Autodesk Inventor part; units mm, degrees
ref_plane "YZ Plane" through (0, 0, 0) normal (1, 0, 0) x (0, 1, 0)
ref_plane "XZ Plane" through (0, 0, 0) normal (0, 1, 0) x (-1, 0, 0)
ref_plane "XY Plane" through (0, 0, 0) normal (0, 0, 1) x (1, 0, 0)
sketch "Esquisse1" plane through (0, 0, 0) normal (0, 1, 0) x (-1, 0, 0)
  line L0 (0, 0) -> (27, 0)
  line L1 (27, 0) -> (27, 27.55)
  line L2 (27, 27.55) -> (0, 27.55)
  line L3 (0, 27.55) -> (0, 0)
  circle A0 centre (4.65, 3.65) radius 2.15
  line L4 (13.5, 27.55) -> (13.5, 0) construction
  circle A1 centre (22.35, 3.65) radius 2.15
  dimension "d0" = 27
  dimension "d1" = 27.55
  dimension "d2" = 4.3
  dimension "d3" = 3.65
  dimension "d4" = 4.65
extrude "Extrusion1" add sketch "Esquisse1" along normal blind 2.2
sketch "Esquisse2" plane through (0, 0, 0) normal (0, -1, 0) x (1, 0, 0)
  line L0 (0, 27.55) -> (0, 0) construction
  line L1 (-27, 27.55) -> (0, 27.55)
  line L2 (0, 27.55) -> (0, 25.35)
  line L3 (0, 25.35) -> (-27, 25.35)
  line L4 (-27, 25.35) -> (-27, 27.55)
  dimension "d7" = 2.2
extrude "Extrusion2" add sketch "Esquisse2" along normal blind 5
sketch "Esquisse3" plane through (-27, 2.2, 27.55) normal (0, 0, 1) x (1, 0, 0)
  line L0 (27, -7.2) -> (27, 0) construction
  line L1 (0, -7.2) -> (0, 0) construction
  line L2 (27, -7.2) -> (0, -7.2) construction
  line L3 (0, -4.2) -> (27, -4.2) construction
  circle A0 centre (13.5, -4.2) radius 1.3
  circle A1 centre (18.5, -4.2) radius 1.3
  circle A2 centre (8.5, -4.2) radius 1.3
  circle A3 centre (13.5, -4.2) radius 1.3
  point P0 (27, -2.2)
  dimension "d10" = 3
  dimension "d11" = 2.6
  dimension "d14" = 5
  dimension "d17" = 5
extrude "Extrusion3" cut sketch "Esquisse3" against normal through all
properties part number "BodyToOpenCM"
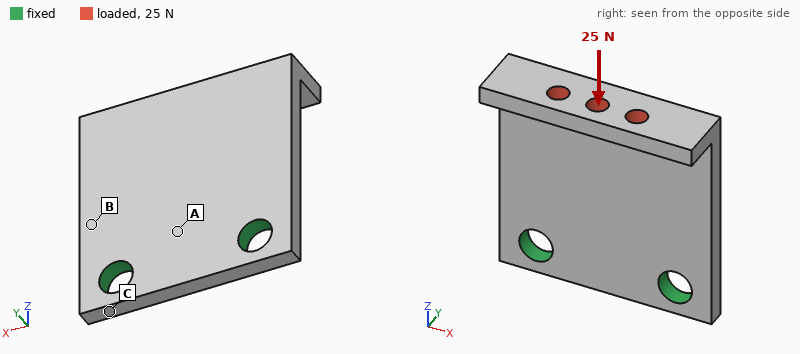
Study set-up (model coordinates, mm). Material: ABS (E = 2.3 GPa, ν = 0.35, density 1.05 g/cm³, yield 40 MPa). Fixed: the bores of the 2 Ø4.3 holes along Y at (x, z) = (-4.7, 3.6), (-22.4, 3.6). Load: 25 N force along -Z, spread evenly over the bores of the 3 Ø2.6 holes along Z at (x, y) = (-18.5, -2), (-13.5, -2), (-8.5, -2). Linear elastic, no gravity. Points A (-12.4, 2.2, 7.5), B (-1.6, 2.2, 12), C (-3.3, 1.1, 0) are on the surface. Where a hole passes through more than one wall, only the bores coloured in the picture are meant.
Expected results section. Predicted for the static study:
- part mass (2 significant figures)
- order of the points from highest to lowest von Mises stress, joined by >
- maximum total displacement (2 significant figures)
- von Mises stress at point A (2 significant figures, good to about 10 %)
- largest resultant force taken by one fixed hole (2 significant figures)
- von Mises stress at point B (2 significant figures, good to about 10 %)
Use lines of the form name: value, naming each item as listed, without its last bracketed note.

part mass: 1.9 g
order of the points from highest to lowest von Mises stress, joined by >: B > A > C
maximum total displacement: 0.41 mm
von Mises stress at point A: 2.3 MPa
largest resultant force taken by one fixed hole: 13 N
von Mises stress at point B: 3.4 MPa
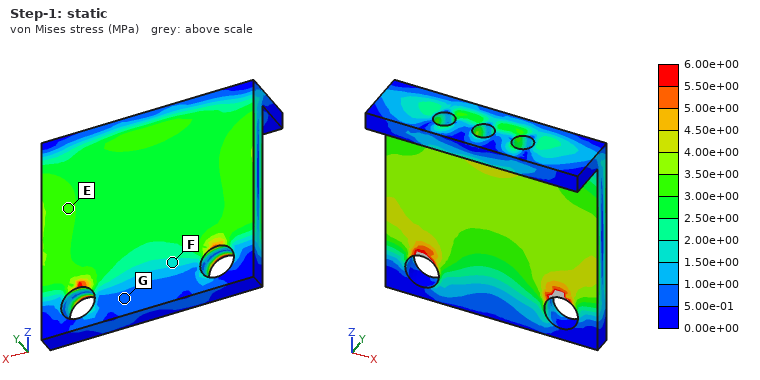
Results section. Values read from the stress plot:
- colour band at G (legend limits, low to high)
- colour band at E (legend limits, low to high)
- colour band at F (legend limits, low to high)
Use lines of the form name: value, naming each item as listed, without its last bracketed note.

colour band at G: 5.00e-01 to 1.00e+00 MPa
colour band at E: 3.00e+00 to 3.50e+00 MPa
colour band at F: 1.50e+00 to 2.00e+00 MPa
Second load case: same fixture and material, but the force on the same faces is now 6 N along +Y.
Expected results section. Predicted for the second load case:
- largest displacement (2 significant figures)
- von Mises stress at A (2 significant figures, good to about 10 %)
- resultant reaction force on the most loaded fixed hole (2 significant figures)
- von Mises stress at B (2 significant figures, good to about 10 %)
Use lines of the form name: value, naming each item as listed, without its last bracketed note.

largest displacement: 0.42 mm
von Mises stress at A: 3.4 MPa
resultant reaction force on the most loaded fixed hole: 3.0 N
von Mises stress at B: 4.2 MPa
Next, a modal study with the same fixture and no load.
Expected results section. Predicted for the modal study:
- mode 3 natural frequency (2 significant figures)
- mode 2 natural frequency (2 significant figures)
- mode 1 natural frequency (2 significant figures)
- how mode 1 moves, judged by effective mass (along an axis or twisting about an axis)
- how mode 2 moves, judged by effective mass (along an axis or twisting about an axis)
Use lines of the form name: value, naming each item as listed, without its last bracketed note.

mode 3 natural frequency: 4500 Hz
mode 2 natural frequency: 1700 Hz
mode 1 natural frequency: 780 Hz
how mode 1 moves, judged by effective mass: along Y
how mode 2 moves, judged by effective mass: twisting about Z
